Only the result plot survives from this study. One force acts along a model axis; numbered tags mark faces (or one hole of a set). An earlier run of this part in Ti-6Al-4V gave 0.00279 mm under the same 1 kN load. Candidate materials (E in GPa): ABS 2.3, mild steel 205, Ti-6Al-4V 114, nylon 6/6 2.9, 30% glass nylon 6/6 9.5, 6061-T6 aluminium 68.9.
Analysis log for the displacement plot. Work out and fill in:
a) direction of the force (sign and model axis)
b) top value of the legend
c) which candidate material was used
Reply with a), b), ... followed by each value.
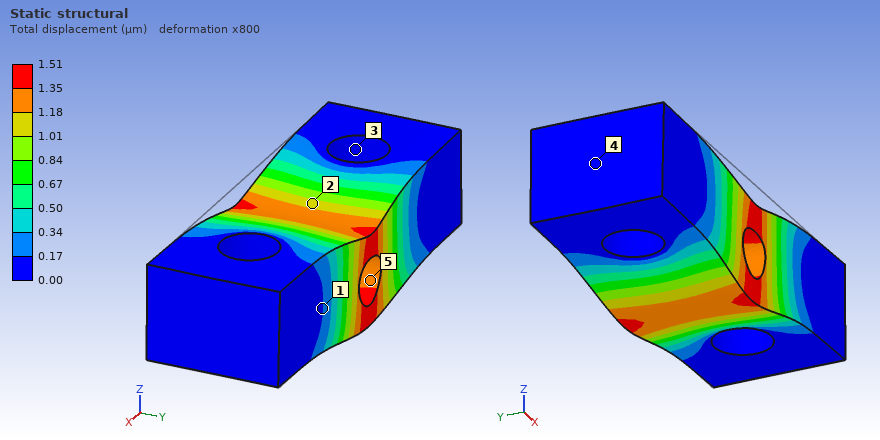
a) -Z
b) 1.51 µm
c) mild steel
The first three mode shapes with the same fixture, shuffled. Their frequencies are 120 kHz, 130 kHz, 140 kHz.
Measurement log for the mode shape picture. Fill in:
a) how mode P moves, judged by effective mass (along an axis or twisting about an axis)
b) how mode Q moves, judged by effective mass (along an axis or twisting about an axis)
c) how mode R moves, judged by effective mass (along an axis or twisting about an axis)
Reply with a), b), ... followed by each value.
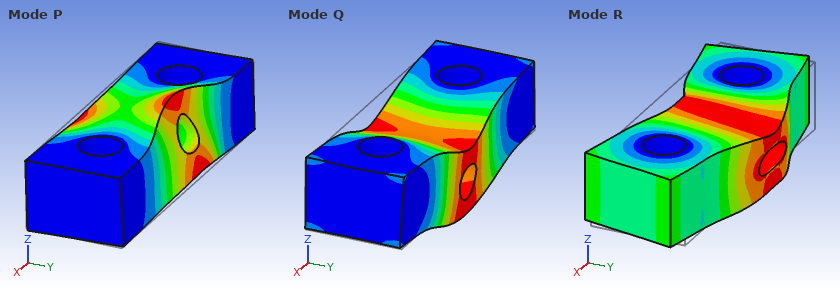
a) twisting about X
b) along Z
c) along Y
